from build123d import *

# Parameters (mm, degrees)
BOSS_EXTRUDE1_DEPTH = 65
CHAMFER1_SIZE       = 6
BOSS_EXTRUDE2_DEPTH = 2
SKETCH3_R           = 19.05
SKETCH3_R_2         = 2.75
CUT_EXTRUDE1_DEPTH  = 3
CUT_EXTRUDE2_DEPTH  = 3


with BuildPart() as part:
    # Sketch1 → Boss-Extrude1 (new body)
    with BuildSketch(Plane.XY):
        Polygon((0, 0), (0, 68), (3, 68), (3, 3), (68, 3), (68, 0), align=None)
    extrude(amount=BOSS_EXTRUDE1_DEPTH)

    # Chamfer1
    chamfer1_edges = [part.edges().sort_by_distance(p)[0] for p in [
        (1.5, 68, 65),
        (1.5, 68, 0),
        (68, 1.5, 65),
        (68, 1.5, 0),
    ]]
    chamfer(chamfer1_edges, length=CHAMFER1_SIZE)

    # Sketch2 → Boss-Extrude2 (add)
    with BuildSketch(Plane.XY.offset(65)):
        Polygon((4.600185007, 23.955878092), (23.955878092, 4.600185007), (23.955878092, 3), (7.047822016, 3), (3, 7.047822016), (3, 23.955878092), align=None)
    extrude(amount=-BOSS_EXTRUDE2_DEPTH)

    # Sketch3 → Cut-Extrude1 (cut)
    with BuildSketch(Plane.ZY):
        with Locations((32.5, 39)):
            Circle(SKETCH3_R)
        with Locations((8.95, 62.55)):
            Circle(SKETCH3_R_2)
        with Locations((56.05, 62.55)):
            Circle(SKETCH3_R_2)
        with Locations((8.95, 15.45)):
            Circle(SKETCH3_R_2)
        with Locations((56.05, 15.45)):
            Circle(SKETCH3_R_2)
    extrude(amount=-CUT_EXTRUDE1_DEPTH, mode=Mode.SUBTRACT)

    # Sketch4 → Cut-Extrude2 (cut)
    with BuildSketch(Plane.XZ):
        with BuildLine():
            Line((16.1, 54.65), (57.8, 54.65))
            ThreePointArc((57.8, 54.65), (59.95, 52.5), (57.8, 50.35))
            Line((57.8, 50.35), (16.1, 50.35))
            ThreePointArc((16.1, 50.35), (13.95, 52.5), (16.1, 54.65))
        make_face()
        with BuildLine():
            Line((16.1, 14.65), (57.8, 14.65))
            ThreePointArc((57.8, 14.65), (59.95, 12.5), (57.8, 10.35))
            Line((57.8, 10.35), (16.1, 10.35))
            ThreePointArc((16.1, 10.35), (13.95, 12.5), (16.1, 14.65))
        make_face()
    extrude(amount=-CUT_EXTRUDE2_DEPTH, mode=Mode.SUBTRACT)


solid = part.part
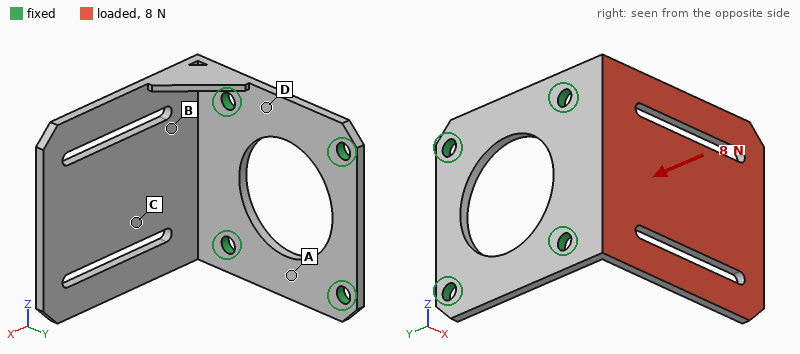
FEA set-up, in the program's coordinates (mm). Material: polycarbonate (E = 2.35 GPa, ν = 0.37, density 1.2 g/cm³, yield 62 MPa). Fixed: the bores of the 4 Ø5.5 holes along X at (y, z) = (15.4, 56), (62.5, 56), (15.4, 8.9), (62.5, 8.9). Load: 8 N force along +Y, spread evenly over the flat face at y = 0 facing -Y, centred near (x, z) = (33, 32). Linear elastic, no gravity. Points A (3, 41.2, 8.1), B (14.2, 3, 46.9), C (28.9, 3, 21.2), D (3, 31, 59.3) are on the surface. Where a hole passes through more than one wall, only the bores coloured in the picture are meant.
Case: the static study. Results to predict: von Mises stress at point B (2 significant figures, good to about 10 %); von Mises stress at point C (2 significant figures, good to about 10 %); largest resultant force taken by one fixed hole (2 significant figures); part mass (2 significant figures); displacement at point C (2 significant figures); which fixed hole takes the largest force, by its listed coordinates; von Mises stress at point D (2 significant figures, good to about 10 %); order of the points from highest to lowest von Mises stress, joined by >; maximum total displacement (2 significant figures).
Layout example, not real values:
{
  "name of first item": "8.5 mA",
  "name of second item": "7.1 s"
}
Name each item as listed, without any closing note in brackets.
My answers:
{
  "von Mises stress at point B": "1.7 MPa",
  "von Mises stress at point C": "0.85 MPa",
  "largest resultant force taken by one fixed hole": "4.9 N",
  "part mass": "26 g",
  "displacement at point C": "0.34 mm",
  "which fixed hole takes the largest force, by its listed coordinates": "(15.4, 8.9)",
  "von Mises stress at point D": "0.60 MPa",
  "order of the points from highest to lowest von Mises stress, joined by >": "B > C > D > A",
  "maximum total displacement": "1.1 mm"
}
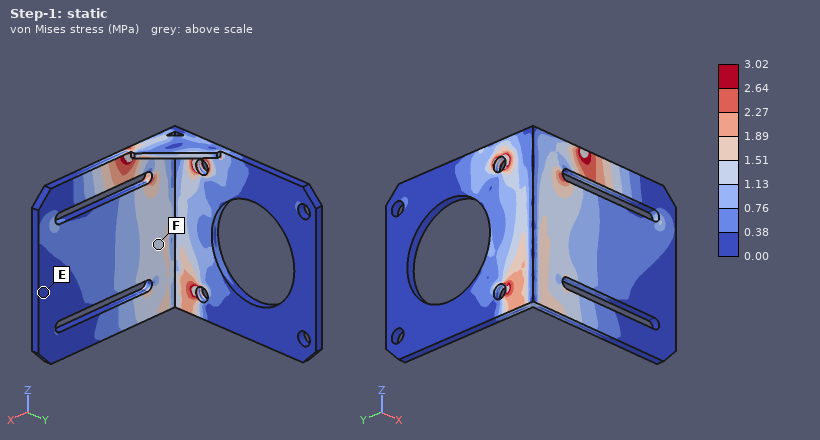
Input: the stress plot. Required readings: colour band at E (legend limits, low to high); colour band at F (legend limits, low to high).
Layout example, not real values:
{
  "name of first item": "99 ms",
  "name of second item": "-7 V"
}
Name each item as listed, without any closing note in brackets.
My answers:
{
  "colour band at E": "0.00 to 0.38 MPa",
  "colour band at F": "1.13 to 1.51 MPa"
}
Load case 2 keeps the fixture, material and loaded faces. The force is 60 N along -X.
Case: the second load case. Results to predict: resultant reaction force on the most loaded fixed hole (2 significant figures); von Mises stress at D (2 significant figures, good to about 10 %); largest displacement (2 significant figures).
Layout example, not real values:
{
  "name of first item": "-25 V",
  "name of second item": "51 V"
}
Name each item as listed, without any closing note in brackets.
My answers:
{
  "resultant reaction force on the most loaded fixed hole": "32 N",
  "von Mises stress at D": "1.4 MPa",
  "largest displacement": "1.3 mm"
}
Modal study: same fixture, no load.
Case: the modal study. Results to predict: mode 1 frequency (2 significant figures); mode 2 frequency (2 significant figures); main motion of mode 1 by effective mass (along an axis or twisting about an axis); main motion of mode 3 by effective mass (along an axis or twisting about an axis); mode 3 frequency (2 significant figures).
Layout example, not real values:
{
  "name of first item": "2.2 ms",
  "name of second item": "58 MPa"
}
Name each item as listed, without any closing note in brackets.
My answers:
{
  "mode 1 frequency": "150 Hz",
  "mode 2 frequency": "380 Hz",
  "main motion of mode 1 by effective mass": "along Y",
  "main motion of mode 3 by effective mass": "along Z",
  "mode 3 frequency": "620 Hz"
}
